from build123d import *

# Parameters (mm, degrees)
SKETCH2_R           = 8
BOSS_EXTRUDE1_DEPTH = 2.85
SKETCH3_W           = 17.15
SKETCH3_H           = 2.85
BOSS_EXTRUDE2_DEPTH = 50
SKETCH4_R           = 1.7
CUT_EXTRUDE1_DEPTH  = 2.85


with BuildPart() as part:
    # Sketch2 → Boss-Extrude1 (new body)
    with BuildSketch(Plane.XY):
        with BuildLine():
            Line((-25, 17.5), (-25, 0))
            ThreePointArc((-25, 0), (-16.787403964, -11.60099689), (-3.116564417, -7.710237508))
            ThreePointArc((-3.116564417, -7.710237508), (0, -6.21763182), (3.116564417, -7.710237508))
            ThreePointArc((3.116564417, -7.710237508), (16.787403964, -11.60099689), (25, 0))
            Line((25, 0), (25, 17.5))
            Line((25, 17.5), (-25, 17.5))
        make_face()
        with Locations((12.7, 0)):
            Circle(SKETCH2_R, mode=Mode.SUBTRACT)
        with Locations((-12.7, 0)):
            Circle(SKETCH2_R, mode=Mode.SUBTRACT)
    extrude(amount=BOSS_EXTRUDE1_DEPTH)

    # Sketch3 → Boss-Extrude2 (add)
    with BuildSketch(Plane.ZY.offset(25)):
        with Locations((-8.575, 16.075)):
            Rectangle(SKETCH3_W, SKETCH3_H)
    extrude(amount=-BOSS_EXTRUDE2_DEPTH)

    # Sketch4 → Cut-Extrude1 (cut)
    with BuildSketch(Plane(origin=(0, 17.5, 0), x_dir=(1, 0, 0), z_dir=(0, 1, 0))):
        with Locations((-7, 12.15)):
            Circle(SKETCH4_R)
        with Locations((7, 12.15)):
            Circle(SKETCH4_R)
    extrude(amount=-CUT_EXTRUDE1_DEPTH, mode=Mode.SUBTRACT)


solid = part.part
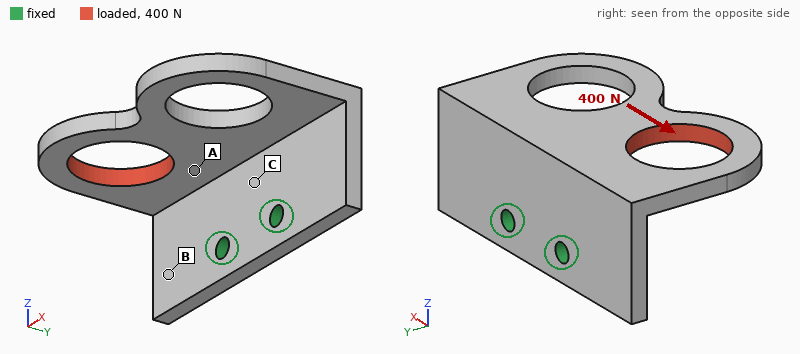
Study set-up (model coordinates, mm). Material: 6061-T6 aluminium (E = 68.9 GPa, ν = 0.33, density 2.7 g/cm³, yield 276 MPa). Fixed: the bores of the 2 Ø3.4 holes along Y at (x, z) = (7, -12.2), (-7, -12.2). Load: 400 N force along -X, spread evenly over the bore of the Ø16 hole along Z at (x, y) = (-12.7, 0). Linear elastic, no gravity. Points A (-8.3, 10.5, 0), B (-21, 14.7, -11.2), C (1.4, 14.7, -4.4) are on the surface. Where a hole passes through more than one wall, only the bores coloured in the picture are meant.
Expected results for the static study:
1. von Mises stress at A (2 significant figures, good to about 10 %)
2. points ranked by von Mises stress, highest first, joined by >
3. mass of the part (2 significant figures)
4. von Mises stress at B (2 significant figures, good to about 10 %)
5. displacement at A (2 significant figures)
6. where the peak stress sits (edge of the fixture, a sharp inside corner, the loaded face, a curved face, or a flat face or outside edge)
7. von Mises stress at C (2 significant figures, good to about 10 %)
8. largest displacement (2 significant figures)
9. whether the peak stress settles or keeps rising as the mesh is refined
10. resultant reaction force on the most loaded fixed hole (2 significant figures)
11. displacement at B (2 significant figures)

46 MPa
C > A > B
14 g
20 MPa
0.051 mm
edge of the fixture
69 MPa
0.19 mm
keeps rising
480 N
0.042 mm
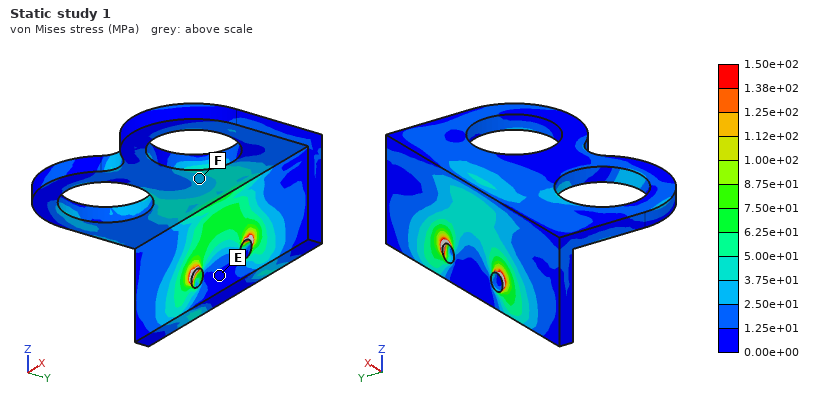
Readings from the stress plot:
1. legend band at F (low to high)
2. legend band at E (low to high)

2.50e+01 to 3.75e+01 MPa
0.00e+00 to 1.25e+01 MPa
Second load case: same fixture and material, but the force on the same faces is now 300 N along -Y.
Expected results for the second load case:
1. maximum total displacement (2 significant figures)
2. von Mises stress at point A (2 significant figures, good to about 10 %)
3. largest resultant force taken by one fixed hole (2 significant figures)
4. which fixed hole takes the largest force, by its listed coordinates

0.22 mm
22 MPa
330 N
(-7, -12.2)
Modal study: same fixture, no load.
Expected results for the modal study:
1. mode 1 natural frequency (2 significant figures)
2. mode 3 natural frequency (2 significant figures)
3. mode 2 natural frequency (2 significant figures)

2100 Hz
4700 Hz
2900 Hz
